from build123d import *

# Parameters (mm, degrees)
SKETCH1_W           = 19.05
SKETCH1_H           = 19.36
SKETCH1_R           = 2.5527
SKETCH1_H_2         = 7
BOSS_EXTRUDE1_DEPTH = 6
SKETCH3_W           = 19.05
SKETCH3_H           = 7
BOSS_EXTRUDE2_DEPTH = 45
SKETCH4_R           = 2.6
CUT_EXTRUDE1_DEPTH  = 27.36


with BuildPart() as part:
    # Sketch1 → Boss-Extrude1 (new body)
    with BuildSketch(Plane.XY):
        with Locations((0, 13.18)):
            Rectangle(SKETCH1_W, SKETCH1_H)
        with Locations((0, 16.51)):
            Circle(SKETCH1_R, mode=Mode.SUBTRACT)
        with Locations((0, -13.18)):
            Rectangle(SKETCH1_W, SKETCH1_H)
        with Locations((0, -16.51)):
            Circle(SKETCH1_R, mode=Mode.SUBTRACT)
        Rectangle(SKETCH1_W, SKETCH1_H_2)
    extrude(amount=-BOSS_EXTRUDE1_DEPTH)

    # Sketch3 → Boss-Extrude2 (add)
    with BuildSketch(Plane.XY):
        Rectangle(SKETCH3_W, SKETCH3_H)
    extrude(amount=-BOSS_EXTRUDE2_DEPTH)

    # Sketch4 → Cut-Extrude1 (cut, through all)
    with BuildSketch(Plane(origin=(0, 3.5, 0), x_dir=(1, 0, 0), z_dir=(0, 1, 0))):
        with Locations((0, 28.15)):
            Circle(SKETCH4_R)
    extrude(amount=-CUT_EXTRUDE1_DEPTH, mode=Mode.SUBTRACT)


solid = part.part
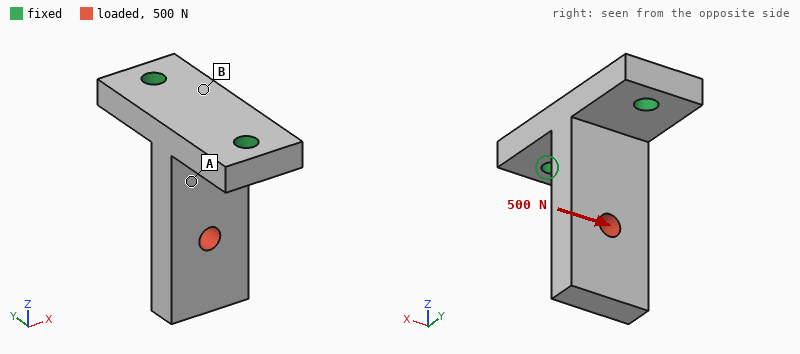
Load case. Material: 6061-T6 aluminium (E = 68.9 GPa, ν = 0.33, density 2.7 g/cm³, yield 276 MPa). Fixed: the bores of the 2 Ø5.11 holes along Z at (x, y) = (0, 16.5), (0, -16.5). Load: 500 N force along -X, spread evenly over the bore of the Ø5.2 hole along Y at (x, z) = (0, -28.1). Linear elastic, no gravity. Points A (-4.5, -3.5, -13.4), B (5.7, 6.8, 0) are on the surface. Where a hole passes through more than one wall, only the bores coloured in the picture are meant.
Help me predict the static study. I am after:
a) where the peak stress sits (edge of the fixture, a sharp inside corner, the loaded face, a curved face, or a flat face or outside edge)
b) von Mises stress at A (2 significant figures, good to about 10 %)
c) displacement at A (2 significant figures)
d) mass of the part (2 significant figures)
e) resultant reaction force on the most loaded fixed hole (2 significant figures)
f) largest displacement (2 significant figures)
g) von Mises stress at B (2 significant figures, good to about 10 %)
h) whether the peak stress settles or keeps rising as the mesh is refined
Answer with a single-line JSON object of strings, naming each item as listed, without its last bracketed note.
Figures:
{"where the peak stress sits": "edge of the fixture", "von Mises stress at A": "11 MPa", "displacement at A": "0.031 mm", "mass of the part": "27 g", "resultant reaction force on the most loaded fixed hole": "250 N", "largest displacement": "0.12 mm", "von Mises stress at B": "29 MPa", "whether the peak stress settles or keeps rising as the mesh is refined": "keeps rising"}
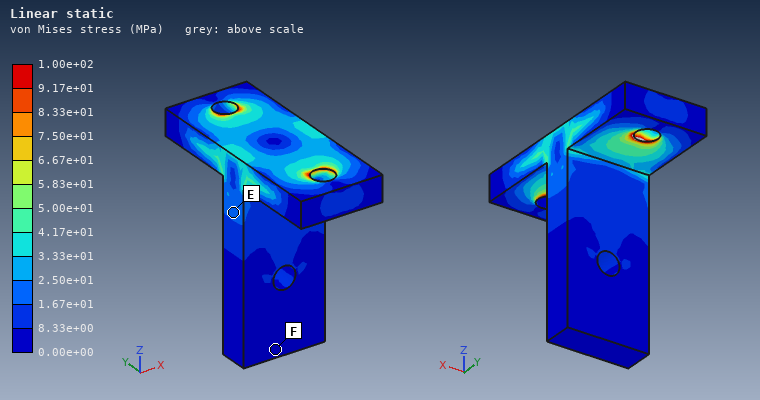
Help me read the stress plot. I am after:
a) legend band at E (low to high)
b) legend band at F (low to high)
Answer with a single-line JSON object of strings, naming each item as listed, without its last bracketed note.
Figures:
{"legend band at E": "1.67e+01 to 2.50e+01 MPa", "legend band at F": "0.00e+00 to 8.33e+00 MPa"}
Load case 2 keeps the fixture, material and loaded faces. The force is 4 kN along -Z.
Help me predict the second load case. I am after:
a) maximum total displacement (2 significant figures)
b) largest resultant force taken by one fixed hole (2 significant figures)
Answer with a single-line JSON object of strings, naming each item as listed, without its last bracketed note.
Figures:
{"maximum total displacement": "45 µm", "largest resultant force taken by one fixed hole": "2.0 kN"}
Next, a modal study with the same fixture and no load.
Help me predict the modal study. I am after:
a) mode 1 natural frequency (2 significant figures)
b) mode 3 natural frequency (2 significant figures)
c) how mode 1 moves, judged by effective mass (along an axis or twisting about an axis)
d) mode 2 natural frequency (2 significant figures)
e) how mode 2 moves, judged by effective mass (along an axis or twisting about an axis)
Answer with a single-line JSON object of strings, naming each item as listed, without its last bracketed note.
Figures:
{"mode 1 natural frequency": "3100 Hz", "mode 3 natural frequency": "12 kHz", "how mode 1 moves, judged by effective mass": "along Y", "mode 2 natural frequency": "3500 Hz", "how mode 2 moves, judged by effective mass": "along X"}
